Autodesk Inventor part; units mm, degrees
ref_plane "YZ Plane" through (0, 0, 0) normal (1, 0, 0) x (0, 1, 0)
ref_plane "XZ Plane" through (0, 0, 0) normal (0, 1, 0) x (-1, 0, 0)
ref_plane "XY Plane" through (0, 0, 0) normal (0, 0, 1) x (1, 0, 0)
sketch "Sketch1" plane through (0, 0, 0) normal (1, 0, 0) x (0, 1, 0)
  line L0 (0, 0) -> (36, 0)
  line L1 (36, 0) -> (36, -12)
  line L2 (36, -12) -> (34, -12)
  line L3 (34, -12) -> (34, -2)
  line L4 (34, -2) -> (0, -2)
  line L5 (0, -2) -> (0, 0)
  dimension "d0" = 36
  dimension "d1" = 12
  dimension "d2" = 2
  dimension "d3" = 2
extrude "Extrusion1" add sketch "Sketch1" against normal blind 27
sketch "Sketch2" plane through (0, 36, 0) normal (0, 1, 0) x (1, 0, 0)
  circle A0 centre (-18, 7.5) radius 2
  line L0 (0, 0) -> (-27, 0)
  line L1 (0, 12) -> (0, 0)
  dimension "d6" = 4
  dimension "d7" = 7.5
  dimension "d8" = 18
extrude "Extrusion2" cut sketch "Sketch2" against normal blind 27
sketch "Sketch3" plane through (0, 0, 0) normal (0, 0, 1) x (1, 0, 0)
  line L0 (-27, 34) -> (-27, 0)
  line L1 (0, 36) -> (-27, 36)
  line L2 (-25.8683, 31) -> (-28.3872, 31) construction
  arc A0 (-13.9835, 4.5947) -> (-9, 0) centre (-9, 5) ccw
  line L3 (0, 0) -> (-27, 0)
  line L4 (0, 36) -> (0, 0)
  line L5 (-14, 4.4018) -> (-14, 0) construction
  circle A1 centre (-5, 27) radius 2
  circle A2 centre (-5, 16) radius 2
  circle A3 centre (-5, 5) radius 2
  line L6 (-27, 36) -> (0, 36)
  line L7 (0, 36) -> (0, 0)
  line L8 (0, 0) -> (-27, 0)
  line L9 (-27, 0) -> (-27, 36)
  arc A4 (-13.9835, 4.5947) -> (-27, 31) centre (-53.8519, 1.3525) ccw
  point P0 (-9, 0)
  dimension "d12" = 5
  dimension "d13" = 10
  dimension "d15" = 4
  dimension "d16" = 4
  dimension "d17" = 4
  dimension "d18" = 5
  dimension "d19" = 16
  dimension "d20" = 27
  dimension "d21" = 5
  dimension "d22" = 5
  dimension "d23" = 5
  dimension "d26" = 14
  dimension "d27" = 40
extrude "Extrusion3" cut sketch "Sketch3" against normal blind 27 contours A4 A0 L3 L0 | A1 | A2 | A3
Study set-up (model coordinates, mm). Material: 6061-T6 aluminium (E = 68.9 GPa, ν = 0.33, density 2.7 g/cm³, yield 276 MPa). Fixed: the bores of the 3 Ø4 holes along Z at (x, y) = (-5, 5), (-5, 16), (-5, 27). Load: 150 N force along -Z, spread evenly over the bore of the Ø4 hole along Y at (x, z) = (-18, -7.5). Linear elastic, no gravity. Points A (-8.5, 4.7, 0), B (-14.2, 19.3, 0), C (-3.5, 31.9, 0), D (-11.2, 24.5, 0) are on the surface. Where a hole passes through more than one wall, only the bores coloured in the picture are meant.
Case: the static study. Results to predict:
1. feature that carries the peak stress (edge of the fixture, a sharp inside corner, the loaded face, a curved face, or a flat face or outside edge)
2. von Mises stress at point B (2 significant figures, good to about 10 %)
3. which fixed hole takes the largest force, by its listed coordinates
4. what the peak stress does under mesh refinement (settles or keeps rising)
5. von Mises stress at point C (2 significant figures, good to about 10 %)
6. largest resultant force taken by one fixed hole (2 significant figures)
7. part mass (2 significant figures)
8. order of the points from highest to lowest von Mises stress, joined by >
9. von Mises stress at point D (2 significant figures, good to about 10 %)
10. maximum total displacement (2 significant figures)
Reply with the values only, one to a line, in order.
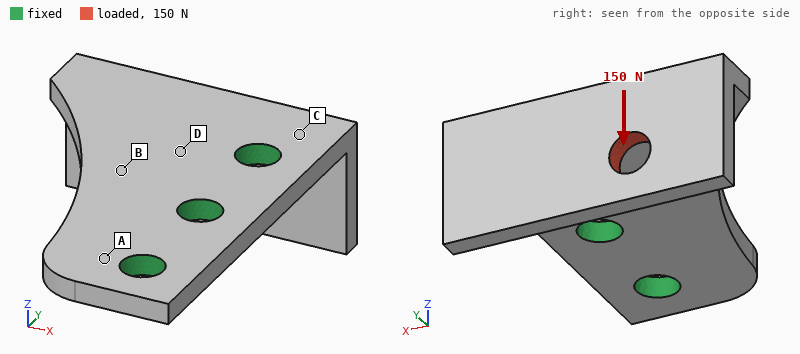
edge of the fixture
46 MPa
(-5, 27)
keeps rising
110 MPa
180 N
4.9 g
C > D > B > A
75 MPa
0.25 mm
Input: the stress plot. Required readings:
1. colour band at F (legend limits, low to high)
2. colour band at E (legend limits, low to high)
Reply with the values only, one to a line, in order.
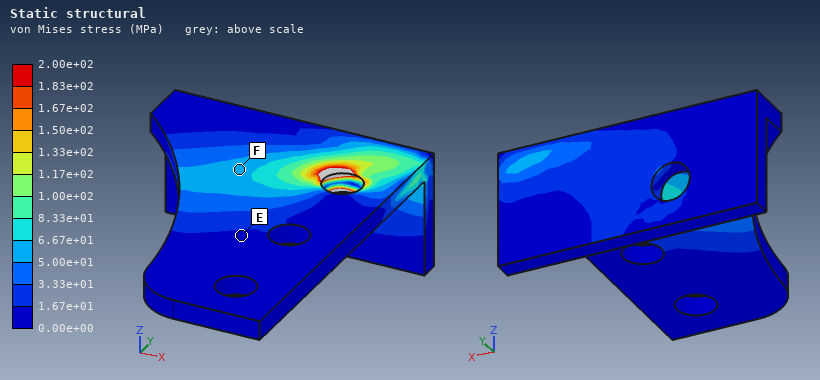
5.00e+01 to 6.67e+01 MPa
0.00e+00 to 1.67e+01 MPa
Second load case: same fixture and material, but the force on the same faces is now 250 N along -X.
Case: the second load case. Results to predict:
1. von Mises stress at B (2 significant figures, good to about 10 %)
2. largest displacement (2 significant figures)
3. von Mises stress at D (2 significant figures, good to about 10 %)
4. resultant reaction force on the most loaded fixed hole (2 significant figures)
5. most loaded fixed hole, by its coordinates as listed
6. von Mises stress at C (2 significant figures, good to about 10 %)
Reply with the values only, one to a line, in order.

41 MPa
0.19 mm
53 MPa
330 N
(-5, 27)
72 MPa
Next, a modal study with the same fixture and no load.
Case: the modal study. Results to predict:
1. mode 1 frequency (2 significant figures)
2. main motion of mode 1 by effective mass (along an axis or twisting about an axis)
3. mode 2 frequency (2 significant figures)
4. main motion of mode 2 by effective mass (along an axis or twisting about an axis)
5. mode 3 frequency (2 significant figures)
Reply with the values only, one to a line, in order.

3700 Hz
along Z
6500 Hz
along Y
12 kHz
